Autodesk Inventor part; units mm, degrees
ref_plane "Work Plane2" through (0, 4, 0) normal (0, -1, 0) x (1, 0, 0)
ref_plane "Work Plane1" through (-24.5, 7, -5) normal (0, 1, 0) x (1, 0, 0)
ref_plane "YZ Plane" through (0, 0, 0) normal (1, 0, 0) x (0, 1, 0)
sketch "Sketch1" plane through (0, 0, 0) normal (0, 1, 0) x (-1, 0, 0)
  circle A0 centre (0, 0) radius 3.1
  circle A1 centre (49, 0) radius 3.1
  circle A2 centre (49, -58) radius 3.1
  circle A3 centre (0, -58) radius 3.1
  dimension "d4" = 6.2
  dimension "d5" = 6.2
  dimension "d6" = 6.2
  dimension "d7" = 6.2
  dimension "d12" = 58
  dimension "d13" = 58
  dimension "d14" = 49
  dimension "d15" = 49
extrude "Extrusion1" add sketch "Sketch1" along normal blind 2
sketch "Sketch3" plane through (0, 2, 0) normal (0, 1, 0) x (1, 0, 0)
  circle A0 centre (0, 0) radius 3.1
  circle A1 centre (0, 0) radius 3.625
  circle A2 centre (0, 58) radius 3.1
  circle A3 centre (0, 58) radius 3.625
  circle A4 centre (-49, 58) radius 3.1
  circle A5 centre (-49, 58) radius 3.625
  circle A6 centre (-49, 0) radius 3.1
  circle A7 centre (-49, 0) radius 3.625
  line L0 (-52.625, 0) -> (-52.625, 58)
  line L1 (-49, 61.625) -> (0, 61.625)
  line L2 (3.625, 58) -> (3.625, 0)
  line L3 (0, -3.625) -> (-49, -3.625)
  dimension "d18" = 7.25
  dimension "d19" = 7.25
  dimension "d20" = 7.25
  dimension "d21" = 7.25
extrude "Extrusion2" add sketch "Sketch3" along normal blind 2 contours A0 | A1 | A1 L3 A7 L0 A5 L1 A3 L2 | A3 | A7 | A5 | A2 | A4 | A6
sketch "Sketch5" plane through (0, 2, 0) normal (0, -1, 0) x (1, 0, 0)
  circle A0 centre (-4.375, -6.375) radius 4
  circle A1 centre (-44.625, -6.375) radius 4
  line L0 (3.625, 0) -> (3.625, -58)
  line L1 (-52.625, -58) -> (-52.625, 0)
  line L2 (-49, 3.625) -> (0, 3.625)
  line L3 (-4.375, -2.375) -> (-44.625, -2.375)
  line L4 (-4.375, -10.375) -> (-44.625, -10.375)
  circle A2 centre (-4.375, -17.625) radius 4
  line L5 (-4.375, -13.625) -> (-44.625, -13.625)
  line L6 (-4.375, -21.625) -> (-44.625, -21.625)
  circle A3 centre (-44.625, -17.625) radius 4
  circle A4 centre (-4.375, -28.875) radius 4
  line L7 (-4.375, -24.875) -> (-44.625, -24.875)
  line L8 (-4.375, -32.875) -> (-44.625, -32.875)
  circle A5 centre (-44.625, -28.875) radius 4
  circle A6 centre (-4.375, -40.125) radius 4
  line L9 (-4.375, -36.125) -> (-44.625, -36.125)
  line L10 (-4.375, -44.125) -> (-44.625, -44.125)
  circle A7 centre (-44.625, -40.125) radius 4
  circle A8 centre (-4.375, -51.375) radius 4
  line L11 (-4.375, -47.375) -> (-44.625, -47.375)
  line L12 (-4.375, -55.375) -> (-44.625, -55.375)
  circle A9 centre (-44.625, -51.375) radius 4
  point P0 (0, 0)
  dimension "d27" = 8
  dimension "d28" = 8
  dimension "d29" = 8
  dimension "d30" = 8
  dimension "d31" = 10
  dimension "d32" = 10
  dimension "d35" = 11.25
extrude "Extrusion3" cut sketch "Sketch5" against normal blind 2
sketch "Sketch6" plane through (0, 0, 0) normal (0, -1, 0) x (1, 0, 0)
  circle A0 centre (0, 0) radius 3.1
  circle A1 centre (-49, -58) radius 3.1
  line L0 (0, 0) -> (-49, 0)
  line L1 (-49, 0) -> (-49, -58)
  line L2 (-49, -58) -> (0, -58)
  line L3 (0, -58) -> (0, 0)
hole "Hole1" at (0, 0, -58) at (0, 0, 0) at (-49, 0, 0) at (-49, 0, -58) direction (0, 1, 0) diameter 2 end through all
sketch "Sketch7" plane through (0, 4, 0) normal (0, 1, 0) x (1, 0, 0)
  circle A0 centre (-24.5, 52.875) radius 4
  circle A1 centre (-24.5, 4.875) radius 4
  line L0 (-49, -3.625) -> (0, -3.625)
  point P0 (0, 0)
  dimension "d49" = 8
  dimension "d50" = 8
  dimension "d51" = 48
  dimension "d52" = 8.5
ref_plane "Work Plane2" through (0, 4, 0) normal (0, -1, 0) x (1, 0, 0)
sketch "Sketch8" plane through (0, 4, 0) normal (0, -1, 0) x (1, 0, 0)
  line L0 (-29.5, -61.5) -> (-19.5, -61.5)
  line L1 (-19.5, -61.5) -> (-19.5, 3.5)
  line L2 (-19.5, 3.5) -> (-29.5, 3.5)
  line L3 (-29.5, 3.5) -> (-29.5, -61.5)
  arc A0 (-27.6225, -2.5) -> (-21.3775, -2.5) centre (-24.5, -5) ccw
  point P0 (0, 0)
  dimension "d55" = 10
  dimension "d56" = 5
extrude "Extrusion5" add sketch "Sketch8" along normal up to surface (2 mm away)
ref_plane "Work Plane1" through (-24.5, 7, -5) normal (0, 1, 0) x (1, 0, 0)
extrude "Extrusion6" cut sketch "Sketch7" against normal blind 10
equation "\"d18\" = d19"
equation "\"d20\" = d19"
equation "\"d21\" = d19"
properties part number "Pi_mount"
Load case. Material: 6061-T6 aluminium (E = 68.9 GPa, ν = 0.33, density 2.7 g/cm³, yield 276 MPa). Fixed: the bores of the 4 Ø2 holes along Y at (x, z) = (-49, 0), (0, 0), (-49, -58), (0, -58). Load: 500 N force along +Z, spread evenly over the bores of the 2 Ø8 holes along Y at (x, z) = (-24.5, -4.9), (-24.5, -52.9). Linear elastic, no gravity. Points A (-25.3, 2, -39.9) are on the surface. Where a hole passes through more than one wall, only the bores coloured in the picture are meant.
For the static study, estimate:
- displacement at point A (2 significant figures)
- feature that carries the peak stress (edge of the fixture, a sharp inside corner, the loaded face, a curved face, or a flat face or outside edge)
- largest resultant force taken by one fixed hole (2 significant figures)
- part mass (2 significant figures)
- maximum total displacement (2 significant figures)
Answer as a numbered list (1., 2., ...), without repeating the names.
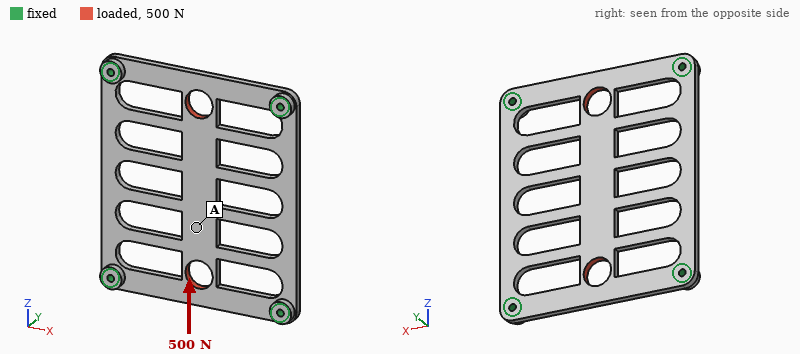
1. 38 µm
2. the loaded face
3. 130 N
4. 12 g
5. 44 µm
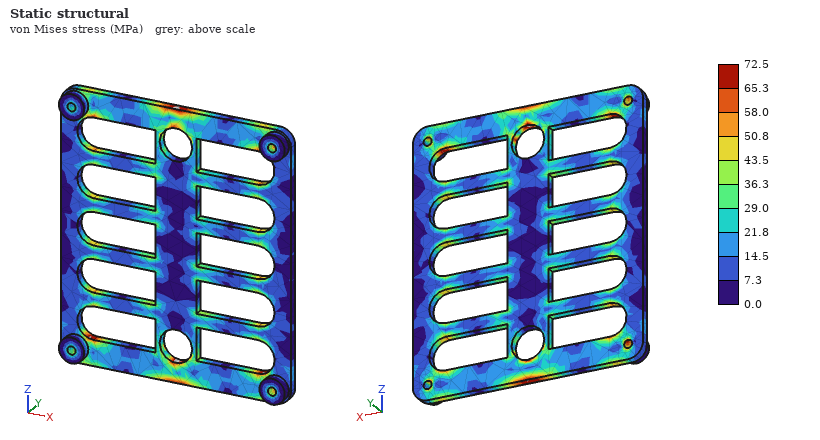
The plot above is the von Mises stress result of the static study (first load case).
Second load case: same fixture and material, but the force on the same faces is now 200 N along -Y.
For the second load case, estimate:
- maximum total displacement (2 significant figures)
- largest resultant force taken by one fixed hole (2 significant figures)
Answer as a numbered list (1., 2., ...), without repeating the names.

1. 0.14 mm
2. 52 N
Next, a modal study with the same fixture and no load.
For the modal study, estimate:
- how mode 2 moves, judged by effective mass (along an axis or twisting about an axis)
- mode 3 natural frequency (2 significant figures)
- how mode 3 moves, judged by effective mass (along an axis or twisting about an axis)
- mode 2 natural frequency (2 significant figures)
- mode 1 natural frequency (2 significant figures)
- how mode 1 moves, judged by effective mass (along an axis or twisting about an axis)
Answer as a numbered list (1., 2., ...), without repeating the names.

1. twisting about Z
2. 4100 Hz
3. twisting about X
4. 3300 Hz
5. 2000 Hz
6. along Y
